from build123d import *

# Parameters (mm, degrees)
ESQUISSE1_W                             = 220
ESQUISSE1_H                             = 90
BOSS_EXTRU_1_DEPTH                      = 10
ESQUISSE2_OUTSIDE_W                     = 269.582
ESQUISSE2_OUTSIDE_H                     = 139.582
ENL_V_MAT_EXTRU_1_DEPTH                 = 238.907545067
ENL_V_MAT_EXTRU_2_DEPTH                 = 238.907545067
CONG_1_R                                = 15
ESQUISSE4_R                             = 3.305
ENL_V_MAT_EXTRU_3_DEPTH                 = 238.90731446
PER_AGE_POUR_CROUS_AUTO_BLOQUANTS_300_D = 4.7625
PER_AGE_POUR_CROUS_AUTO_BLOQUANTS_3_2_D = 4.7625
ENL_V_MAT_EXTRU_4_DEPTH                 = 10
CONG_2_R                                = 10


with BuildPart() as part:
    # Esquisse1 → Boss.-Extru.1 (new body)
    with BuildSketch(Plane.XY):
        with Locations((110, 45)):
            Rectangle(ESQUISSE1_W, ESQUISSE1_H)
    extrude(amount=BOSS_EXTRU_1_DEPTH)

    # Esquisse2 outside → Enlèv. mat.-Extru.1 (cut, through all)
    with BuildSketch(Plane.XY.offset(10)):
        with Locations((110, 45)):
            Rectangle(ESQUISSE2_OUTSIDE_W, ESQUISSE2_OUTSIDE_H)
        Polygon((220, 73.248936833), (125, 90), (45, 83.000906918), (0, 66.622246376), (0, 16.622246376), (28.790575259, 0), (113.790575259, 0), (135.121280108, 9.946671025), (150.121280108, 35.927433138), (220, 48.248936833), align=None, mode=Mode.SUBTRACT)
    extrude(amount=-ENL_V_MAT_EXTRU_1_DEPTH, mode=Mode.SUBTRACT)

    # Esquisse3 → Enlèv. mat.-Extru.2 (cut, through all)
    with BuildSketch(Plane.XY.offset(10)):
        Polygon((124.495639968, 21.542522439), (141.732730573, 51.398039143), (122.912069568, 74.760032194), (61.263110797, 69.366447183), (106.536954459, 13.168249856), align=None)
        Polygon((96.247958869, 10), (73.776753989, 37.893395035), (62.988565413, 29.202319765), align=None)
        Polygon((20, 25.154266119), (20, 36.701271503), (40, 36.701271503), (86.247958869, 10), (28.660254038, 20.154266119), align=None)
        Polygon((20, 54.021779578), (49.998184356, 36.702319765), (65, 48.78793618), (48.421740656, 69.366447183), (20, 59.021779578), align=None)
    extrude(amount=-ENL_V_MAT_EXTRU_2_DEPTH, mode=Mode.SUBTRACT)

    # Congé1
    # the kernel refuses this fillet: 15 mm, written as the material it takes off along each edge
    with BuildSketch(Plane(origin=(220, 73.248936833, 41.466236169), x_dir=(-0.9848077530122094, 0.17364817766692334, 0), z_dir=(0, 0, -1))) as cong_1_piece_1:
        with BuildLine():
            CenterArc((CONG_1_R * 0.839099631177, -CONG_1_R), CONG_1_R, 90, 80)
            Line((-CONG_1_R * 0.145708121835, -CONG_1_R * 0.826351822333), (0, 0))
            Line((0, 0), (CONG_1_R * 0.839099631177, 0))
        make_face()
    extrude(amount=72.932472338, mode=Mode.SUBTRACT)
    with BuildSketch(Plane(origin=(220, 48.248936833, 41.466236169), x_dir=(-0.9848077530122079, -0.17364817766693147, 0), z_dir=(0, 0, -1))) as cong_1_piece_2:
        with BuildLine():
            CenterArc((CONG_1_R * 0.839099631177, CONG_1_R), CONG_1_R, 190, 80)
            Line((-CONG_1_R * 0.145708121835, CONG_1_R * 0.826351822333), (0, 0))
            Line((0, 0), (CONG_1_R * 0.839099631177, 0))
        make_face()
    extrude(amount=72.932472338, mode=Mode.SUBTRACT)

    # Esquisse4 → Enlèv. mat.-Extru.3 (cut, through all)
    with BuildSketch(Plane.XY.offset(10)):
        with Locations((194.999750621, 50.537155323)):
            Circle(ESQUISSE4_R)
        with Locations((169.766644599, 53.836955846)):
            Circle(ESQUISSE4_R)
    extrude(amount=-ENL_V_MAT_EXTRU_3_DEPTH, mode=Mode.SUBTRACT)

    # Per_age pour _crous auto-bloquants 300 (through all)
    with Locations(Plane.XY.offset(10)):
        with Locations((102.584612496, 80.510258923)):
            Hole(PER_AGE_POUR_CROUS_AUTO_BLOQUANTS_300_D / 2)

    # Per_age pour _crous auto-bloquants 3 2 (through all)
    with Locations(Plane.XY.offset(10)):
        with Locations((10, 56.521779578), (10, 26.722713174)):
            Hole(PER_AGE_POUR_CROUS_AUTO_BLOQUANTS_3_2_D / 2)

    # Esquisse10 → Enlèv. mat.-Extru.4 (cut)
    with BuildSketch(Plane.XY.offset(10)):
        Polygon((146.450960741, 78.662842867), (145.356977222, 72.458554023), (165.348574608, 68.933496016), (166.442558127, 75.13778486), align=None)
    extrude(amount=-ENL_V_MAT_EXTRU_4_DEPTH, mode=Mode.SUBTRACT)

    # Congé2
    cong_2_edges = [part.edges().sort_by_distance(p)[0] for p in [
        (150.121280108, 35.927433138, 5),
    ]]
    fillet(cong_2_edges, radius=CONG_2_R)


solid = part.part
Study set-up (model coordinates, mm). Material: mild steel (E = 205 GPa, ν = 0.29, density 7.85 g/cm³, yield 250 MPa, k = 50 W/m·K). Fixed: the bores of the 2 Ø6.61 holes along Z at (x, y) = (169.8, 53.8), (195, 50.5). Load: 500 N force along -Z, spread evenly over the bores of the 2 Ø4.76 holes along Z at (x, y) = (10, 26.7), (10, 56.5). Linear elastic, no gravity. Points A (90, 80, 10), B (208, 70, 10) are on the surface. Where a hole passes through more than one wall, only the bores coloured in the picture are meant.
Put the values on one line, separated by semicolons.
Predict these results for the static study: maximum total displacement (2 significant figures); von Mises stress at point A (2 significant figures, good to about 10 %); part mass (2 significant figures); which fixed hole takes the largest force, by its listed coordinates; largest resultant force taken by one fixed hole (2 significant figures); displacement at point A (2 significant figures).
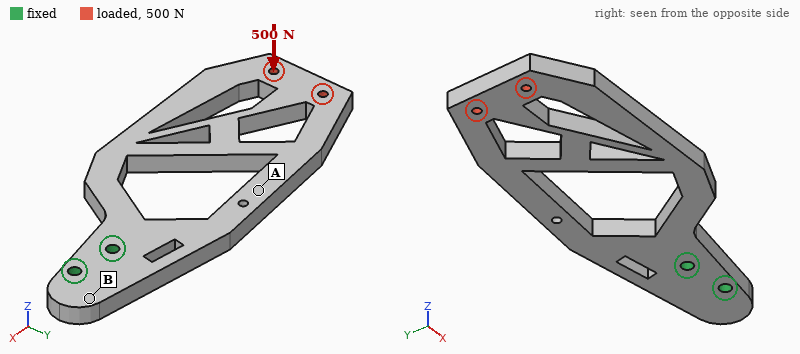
1.4 mm; 84 MPa; 740 g; (169.8, 53.8); 1.6 kN; 0.36 mm
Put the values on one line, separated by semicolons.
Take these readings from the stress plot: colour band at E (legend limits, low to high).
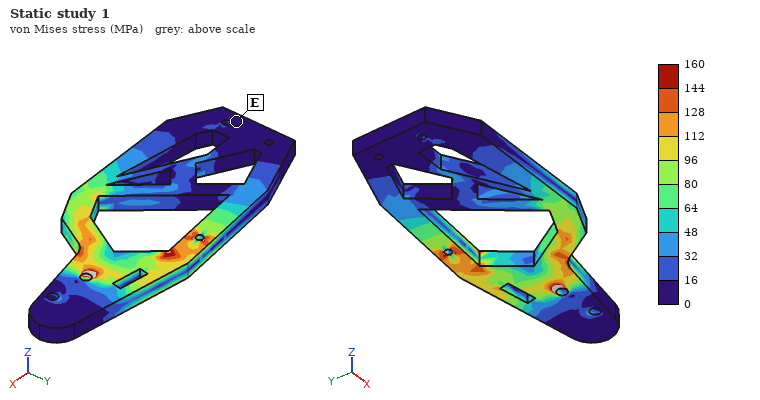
0 to 16 MPa
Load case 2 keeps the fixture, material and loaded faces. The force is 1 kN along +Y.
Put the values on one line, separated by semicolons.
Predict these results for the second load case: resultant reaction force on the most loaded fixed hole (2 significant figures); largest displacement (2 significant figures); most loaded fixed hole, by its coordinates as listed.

5.7 kN; 0.24 mm; (169.8, 53.8)
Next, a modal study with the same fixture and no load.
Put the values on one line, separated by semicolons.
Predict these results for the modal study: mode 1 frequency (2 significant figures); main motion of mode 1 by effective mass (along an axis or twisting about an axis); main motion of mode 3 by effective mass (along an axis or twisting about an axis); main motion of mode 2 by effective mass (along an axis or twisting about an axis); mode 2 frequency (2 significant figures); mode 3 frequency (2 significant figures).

220 Hz; along Z; twisting about X; along Y; 650 Hz; 780 Hz
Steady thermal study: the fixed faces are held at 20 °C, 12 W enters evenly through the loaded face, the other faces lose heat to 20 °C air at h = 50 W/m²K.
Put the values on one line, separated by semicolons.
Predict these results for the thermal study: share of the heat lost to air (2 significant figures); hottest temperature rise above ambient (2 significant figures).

95 %; 27 K
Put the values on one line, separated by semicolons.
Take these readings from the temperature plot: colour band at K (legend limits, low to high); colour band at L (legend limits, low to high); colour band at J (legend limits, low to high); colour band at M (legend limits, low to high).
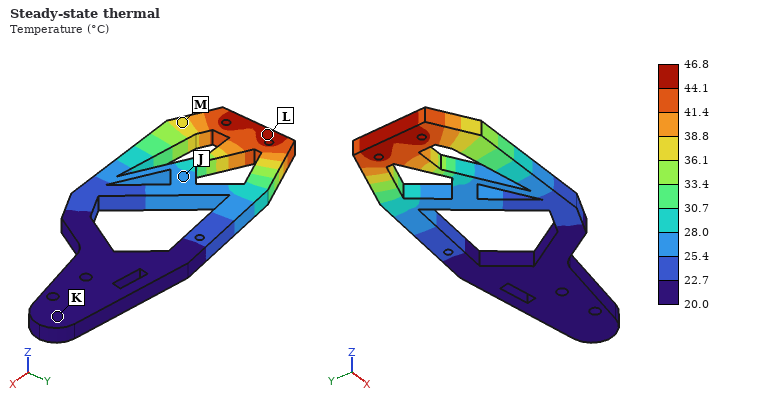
20.0 to 22.7 °C; 44.1 to 46.8 °C; 25.4 to 28.0 °C; 36.1 to 38.8 °C
